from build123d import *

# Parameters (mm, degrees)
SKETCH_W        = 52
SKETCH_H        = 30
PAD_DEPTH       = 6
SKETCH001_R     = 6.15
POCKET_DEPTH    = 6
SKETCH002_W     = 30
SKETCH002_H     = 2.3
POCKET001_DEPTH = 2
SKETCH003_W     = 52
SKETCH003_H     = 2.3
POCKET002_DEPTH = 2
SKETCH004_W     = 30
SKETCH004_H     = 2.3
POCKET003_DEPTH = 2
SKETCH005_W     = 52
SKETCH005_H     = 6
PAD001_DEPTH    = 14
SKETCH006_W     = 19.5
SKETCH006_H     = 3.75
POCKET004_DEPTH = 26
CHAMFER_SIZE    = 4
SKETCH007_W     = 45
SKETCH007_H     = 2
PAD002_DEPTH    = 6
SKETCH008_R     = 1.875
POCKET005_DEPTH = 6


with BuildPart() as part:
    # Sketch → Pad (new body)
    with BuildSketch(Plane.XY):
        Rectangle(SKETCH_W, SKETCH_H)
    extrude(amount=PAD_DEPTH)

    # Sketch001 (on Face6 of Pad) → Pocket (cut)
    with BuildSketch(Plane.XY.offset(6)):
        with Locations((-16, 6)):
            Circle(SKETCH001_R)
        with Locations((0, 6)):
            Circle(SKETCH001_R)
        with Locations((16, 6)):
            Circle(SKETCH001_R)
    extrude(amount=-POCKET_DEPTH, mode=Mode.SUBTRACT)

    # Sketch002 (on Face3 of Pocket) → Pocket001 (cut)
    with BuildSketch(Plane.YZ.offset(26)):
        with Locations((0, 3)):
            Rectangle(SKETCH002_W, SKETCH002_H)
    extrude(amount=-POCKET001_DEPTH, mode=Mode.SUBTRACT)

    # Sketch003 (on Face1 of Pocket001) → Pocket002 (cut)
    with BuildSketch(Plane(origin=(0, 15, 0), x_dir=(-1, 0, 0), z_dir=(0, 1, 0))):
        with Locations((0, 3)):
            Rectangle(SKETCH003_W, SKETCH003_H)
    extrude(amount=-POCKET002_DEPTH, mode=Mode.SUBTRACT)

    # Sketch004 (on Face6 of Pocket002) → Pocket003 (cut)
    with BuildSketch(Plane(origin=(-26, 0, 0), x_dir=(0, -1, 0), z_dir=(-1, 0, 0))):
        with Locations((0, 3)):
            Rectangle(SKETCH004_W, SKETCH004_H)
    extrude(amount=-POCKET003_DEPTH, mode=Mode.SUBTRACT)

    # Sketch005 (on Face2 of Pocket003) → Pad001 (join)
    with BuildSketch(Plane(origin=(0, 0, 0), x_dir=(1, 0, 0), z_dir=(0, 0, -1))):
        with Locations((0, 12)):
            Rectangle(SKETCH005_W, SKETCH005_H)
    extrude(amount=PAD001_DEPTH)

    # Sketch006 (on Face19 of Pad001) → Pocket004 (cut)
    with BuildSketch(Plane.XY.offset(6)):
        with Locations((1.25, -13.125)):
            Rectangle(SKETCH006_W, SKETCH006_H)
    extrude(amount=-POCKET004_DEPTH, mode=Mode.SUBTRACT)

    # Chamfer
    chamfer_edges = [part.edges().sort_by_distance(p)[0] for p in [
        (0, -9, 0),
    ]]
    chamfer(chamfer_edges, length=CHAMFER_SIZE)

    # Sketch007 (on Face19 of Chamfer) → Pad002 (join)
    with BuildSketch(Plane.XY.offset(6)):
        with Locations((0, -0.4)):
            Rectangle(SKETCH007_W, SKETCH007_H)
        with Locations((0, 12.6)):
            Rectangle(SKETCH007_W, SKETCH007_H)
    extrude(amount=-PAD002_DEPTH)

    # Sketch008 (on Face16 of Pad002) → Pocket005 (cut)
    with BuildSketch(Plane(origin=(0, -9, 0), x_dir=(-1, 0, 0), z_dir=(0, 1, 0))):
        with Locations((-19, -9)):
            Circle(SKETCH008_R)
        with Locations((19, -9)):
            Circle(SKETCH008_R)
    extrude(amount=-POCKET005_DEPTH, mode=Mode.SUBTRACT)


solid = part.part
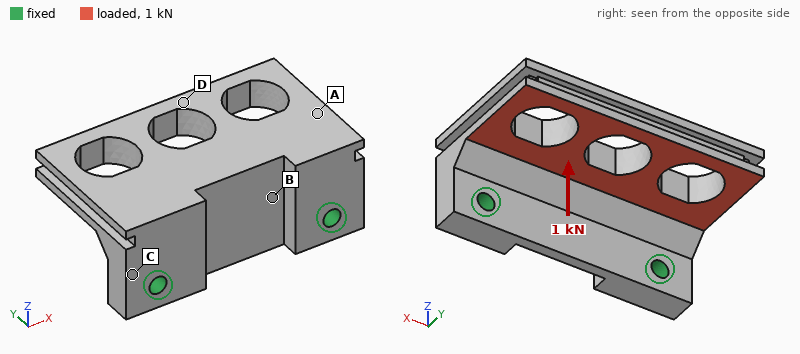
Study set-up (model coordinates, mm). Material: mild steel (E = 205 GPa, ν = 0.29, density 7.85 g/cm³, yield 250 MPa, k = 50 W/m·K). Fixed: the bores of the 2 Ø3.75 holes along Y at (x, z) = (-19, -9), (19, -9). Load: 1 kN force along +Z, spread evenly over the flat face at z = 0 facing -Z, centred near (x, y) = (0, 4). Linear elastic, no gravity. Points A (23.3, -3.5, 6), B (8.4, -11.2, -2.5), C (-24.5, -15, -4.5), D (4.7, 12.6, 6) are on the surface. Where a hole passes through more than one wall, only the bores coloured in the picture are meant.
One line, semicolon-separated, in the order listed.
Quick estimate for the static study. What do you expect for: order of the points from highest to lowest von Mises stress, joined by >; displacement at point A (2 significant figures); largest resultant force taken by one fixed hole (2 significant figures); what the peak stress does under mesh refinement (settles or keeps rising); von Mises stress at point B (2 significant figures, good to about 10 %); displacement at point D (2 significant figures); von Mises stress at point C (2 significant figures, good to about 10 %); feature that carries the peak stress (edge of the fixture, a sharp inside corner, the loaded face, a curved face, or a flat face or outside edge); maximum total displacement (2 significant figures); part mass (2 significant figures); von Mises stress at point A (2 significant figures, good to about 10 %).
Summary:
C > A > B > D; 17 µm; 570 N; keeps rising; 21 MPa; 46 µm; 61 MPa; edge of the fixture; 51 µm; 79 g; 38 MPa
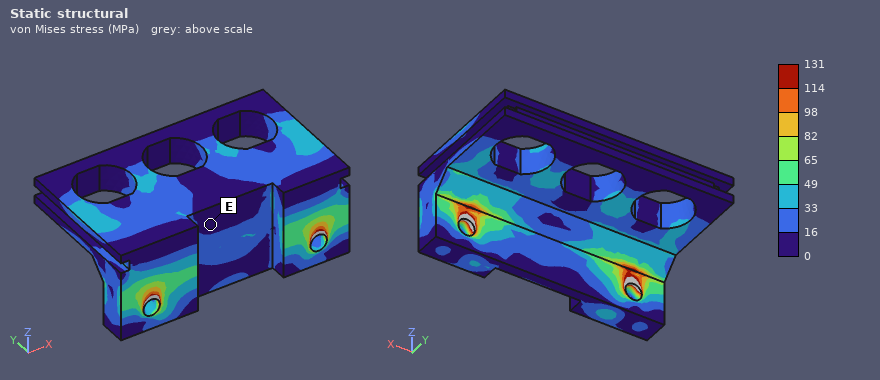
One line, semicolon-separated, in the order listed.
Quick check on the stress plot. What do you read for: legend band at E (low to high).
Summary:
0 to 16 MPa
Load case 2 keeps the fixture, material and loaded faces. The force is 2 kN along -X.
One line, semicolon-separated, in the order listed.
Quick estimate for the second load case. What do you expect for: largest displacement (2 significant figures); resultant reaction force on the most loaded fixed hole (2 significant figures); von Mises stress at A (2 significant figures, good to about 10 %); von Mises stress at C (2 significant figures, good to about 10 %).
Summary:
28 µm; 1.3 kN; 23 MPa; 26 MPa
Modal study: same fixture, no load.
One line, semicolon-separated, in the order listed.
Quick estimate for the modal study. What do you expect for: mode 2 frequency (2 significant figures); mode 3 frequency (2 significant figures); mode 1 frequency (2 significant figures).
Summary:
7700 Hz; 13 kHz; 4600 Hz
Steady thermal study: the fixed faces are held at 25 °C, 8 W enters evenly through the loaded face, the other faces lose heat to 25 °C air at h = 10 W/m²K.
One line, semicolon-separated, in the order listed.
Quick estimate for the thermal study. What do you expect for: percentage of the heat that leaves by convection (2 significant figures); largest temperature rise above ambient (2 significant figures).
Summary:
6.5 %; 21 K
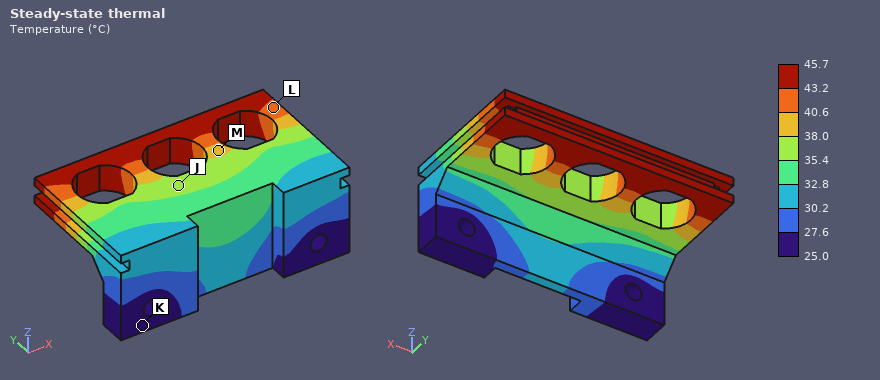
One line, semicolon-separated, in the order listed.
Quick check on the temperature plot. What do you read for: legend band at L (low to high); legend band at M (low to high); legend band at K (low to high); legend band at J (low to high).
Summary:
40.6 to 43.2 °C; 38.0 to 40.6 °C; 25.0 to 27.6 °C; 35.4 to 38.0 °C
